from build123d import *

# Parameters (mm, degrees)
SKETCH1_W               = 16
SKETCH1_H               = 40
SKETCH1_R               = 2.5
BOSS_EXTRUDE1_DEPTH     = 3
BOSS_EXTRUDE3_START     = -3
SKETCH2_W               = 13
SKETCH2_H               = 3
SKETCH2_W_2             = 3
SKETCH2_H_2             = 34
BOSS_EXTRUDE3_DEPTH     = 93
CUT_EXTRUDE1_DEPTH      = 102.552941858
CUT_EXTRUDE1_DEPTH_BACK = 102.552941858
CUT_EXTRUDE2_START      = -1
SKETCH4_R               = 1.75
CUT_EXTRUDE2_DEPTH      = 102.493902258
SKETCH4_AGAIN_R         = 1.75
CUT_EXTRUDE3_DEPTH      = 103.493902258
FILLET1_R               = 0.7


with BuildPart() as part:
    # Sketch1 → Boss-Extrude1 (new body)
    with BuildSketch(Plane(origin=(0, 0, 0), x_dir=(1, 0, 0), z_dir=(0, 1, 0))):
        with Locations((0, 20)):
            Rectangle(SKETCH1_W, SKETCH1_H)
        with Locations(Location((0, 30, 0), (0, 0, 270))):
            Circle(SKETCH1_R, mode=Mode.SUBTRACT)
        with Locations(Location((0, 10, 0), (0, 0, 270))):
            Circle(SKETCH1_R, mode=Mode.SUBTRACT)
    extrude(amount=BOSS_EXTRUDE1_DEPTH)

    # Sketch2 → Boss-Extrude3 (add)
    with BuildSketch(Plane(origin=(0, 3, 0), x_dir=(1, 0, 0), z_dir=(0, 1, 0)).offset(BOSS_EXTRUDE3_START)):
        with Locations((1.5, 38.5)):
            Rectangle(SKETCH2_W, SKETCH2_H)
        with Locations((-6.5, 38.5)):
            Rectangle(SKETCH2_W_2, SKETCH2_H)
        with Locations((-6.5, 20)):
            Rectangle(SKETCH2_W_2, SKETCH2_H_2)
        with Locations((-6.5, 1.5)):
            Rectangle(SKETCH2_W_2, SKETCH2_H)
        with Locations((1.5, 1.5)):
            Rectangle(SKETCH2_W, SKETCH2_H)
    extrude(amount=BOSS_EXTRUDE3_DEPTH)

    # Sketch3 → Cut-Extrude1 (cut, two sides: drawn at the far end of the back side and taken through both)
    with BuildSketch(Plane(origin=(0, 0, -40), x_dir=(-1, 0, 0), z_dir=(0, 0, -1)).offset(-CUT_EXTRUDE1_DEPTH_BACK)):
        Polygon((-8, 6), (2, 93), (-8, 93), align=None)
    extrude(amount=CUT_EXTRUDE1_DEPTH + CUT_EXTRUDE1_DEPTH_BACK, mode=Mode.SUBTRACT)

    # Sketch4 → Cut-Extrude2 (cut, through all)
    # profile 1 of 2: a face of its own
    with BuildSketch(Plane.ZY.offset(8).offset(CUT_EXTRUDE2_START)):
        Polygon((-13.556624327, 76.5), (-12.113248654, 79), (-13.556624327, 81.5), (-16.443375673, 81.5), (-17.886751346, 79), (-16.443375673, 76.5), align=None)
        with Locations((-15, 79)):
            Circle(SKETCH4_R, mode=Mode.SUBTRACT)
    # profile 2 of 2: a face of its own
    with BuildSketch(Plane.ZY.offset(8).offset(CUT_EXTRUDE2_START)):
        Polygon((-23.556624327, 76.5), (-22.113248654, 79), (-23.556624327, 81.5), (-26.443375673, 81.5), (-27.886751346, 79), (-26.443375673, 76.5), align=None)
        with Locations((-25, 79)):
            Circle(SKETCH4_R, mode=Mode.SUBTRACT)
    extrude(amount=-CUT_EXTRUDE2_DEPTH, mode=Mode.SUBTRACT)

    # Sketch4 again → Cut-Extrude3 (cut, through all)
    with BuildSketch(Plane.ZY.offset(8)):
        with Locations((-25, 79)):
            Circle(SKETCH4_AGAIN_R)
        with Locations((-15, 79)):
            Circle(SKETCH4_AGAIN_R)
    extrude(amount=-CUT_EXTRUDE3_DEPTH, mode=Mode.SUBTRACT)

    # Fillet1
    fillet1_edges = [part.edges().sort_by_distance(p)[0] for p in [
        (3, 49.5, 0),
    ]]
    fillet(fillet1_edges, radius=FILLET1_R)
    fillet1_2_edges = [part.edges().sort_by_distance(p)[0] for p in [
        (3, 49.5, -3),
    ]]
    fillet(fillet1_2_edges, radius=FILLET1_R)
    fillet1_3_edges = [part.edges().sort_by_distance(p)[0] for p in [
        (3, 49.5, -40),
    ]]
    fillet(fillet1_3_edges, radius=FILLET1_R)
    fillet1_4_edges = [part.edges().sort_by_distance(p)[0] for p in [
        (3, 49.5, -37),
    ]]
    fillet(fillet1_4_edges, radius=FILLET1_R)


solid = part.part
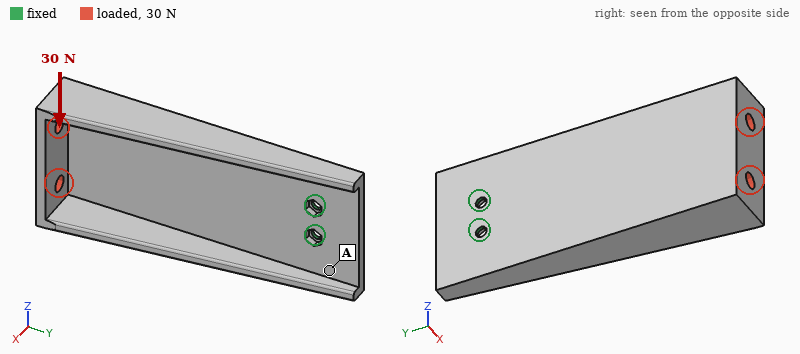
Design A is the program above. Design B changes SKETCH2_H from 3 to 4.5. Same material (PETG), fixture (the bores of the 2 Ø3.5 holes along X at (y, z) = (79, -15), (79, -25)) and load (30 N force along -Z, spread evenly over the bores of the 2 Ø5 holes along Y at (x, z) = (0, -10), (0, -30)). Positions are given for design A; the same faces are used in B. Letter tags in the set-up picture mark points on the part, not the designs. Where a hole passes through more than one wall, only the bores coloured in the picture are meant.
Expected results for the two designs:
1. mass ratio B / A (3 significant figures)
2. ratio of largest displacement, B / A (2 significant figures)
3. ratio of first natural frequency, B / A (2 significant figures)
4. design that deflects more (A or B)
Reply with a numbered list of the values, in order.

1. 1.16
2. 0.82
3. 0.98
4. A
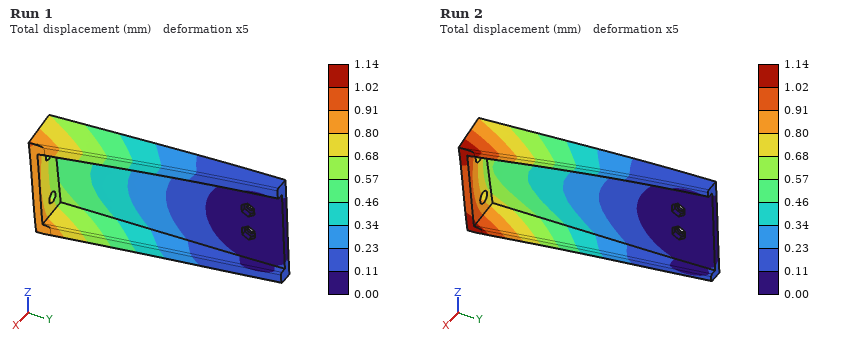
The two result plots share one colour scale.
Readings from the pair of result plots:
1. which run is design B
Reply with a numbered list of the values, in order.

1. Run 1
